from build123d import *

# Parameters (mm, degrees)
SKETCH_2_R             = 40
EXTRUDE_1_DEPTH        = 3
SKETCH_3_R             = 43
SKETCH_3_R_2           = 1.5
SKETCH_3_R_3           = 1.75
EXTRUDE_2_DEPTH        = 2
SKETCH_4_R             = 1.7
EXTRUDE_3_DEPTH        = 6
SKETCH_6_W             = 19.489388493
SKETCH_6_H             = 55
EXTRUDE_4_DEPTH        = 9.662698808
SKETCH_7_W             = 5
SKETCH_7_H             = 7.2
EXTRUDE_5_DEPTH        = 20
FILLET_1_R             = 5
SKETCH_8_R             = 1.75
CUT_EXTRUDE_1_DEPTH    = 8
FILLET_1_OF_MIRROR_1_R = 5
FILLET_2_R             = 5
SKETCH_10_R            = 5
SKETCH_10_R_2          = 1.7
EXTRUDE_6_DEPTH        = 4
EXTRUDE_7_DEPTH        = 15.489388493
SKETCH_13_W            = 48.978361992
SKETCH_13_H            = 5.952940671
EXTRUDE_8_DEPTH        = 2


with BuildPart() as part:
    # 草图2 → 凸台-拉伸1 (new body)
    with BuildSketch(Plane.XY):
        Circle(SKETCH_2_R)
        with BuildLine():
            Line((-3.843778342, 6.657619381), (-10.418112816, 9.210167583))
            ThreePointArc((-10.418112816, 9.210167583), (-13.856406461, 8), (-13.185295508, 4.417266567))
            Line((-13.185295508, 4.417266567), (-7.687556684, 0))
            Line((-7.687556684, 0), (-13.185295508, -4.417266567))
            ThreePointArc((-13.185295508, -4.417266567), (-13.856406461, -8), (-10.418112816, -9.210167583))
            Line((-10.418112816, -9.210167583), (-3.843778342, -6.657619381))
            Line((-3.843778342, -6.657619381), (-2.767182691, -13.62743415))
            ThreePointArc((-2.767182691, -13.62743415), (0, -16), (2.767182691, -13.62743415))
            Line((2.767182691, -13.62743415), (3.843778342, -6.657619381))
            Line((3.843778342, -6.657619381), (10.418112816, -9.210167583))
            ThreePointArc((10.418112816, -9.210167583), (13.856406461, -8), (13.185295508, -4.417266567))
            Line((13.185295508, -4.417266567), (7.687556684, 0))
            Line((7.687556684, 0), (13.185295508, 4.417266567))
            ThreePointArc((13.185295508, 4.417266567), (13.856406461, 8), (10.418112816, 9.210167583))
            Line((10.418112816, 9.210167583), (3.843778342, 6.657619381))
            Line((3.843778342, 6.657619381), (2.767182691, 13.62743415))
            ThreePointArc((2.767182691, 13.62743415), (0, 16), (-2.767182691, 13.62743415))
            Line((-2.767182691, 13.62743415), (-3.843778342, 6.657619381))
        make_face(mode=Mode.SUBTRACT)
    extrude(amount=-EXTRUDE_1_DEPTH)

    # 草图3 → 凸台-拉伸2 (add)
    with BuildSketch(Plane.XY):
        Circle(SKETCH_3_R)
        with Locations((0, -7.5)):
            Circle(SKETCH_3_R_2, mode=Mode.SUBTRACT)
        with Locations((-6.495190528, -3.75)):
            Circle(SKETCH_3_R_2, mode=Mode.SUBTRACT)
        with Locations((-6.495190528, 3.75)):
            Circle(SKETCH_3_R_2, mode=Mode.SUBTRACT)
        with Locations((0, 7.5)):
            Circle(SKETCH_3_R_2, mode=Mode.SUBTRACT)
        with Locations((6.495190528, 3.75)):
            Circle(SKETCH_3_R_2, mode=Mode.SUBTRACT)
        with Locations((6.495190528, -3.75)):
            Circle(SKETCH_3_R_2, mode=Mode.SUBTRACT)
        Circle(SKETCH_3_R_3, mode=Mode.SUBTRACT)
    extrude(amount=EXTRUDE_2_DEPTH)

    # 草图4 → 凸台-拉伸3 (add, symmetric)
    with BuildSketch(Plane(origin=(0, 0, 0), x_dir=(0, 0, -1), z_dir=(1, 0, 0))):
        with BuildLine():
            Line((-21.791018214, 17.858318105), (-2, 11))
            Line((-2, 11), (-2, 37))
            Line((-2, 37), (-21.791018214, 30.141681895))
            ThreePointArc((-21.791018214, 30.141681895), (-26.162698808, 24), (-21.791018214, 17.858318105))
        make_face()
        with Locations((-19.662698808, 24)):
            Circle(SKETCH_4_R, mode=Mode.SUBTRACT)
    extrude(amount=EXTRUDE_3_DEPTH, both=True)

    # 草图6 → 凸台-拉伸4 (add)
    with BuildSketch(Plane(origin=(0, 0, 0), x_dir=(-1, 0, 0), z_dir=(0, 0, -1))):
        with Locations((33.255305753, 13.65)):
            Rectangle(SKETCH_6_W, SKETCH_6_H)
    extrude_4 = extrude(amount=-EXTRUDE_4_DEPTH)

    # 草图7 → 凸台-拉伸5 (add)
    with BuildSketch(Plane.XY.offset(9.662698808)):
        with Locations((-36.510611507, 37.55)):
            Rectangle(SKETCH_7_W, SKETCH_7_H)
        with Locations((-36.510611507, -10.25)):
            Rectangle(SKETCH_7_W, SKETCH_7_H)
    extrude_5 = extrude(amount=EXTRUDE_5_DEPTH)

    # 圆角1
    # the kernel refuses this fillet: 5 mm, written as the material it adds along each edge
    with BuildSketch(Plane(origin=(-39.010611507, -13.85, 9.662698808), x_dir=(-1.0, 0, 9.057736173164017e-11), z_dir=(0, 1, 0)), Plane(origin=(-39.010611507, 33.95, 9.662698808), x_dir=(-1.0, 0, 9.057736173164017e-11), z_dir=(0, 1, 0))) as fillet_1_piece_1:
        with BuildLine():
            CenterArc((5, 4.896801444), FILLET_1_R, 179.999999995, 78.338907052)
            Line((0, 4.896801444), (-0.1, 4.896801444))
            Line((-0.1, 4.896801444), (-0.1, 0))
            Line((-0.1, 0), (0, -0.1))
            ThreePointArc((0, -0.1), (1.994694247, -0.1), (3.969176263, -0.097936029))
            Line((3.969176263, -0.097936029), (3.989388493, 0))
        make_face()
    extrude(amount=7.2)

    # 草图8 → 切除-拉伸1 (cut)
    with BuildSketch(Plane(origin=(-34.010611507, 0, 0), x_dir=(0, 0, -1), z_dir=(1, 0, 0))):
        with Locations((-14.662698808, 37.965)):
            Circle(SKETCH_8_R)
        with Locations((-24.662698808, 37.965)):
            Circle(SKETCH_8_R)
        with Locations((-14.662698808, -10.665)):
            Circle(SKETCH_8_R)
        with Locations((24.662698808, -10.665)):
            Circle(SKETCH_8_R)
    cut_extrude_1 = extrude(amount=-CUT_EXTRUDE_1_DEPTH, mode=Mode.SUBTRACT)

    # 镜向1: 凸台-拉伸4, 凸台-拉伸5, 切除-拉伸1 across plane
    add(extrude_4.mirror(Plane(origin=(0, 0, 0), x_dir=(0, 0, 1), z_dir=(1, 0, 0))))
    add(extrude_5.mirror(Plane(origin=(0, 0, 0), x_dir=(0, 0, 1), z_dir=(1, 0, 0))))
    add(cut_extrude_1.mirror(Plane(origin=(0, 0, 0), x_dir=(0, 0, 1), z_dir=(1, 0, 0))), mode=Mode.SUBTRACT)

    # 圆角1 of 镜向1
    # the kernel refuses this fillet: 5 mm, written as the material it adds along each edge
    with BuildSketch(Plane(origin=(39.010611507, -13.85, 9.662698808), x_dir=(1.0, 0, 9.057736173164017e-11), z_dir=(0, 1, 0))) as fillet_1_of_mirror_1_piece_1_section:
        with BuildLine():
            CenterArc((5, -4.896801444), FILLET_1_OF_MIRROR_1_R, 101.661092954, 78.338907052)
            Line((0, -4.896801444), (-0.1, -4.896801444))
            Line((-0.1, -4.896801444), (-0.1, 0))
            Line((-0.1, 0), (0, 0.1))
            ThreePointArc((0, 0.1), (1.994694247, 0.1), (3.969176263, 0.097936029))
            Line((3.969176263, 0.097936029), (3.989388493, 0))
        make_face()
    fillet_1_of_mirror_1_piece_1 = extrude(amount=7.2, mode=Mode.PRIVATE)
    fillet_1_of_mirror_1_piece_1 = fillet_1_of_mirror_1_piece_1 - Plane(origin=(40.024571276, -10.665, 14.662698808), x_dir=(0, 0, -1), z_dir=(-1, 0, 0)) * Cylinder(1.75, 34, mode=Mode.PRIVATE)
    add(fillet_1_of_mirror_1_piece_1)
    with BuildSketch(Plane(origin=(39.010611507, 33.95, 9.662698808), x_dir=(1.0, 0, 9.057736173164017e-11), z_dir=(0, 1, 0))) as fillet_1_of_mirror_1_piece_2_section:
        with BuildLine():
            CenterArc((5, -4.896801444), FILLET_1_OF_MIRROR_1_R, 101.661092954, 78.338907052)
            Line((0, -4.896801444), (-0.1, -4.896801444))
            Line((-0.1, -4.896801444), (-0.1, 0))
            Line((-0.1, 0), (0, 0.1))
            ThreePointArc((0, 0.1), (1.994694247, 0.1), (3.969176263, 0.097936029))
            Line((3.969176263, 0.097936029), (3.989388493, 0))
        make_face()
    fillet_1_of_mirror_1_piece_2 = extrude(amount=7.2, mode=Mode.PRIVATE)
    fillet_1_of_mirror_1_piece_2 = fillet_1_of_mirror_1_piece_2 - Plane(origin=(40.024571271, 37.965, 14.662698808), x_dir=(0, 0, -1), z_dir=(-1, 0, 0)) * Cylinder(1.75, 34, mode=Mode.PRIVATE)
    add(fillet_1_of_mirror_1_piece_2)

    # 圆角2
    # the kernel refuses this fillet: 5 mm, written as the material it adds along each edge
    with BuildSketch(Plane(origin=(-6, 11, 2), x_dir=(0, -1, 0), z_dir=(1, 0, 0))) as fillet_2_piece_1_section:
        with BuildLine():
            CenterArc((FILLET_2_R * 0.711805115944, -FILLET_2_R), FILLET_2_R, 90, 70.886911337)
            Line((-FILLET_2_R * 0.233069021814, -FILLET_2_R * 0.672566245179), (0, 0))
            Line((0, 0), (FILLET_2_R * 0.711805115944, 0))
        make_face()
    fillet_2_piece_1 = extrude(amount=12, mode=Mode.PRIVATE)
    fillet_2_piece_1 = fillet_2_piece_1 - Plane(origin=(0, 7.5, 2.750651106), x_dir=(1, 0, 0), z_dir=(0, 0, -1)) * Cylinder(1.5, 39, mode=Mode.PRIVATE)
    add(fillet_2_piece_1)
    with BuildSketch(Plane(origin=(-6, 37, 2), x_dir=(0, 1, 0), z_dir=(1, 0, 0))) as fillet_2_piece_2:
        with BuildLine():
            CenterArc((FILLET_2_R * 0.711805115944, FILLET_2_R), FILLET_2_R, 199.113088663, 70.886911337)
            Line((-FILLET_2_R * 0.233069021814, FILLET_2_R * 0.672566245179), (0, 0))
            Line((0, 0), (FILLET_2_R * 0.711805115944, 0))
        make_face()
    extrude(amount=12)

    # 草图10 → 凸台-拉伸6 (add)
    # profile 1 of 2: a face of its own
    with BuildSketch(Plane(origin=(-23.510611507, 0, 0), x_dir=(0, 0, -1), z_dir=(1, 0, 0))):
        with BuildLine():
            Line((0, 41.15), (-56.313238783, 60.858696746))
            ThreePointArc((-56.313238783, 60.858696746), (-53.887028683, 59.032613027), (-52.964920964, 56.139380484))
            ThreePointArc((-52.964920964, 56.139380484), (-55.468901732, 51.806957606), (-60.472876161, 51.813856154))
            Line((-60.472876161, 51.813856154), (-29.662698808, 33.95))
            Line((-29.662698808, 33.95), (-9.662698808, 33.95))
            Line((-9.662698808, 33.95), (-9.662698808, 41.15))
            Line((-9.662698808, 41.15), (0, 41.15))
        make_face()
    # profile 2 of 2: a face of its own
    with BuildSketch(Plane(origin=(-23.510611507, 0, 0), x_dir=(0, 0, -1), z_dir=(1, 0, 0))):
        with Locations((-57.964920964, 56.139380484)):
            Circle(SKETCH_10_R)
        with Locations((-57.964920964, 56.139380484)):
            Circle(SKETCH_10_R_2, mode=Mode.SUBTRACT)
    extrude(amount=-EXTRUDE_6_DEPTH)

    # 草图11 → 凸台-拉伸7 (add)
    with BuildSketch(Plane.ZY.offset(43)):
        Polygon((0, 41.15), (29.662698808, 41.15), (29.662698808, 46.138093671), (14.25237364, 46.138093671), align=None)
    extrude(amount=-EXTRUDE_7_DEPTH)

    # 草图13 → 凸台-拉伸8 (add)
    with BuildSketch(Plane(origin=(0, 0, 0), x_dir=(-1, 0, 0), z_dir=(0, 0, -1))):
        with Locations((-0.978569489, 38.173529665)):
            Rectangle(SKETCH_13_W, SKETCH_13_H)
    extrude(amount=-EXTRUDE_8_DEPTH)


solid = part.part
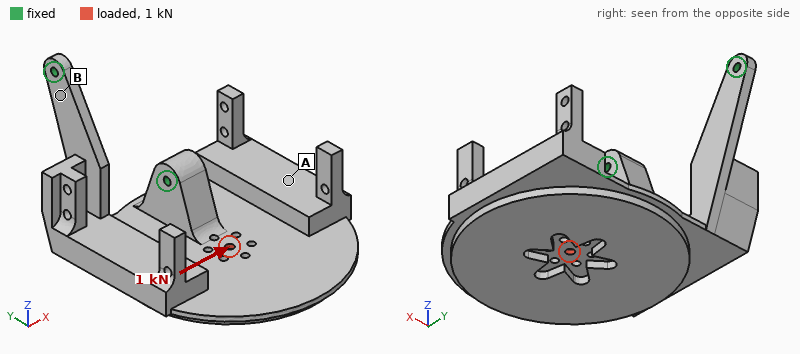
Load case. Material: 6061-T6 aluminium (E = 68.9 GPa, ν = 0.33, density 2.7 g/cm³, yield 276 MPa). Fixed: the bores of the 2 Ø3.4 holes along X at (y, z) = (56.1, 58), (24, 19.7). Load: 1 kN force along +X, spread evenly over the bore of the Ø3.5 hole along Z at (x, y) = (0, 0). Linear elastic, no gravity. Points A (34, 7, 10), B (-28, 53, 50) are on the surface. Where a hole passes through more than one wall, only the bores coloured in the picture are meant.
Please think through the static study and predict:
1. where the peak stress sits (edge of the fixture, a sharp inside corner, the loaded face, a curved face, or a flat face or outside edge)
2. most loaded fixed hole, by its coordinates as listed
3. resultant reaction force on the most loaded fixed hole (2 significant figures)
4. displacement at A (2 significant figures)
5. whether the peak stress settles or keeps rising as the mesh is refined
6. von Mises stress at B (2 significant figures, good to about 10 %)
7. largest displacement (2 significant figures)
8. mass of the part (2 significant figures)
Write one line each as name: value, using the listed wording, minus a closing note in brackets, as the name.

where the peak stress sits: edge of the fixture
most loaded fixed hole, by its coordinates as listed: (24, 19.7)
resultant reaction force on the most loaded fixed hole: 1.0 kN
displacement at A: 0.093 mm
whether the peak stress settles or keeps rising as the mesh is refined: keeps rising
von Mises stress at B: 23 MPa
largest displacement: 0.16 mm
mass of the part: 150 g
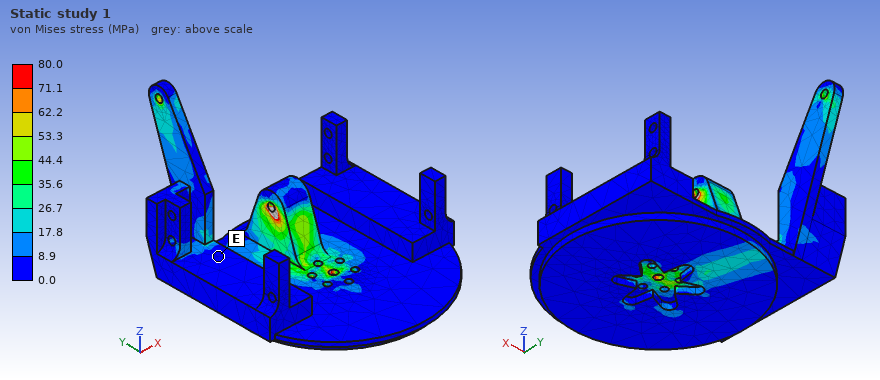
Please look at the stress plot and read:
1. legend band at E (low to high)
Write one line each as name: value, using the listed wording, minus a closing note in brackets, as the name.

legend band at E: 0.0 to 8.9 MPa
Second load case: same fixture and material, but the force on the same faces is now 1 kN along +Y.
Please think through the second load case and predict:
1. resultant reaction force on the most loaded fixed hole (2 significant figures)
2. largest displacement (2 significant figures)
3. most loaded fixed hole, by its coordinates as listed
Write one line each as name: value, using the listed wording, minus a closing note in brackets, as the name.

resultant reaction force on the most loaded fixed hole: 960 N
largest displacement: 93 µm
most loaded fixed hole, by its coordinates as listed: (24, 19.7)
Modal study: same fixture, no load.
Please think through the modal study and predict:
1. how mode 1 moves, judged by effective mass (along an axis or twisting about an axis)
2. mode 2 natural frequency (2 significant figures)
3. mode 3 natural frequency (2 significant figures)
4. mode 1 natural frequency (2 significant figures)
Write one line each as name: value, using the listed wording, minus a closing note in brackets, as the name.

how mode 1 moves, judged by effective mass: along Z
mode 2 natural frequency: 1100 Hz
mode 3 natural frequency: 1300 Hz
mode 1 natural frequency: 1000 Hz
